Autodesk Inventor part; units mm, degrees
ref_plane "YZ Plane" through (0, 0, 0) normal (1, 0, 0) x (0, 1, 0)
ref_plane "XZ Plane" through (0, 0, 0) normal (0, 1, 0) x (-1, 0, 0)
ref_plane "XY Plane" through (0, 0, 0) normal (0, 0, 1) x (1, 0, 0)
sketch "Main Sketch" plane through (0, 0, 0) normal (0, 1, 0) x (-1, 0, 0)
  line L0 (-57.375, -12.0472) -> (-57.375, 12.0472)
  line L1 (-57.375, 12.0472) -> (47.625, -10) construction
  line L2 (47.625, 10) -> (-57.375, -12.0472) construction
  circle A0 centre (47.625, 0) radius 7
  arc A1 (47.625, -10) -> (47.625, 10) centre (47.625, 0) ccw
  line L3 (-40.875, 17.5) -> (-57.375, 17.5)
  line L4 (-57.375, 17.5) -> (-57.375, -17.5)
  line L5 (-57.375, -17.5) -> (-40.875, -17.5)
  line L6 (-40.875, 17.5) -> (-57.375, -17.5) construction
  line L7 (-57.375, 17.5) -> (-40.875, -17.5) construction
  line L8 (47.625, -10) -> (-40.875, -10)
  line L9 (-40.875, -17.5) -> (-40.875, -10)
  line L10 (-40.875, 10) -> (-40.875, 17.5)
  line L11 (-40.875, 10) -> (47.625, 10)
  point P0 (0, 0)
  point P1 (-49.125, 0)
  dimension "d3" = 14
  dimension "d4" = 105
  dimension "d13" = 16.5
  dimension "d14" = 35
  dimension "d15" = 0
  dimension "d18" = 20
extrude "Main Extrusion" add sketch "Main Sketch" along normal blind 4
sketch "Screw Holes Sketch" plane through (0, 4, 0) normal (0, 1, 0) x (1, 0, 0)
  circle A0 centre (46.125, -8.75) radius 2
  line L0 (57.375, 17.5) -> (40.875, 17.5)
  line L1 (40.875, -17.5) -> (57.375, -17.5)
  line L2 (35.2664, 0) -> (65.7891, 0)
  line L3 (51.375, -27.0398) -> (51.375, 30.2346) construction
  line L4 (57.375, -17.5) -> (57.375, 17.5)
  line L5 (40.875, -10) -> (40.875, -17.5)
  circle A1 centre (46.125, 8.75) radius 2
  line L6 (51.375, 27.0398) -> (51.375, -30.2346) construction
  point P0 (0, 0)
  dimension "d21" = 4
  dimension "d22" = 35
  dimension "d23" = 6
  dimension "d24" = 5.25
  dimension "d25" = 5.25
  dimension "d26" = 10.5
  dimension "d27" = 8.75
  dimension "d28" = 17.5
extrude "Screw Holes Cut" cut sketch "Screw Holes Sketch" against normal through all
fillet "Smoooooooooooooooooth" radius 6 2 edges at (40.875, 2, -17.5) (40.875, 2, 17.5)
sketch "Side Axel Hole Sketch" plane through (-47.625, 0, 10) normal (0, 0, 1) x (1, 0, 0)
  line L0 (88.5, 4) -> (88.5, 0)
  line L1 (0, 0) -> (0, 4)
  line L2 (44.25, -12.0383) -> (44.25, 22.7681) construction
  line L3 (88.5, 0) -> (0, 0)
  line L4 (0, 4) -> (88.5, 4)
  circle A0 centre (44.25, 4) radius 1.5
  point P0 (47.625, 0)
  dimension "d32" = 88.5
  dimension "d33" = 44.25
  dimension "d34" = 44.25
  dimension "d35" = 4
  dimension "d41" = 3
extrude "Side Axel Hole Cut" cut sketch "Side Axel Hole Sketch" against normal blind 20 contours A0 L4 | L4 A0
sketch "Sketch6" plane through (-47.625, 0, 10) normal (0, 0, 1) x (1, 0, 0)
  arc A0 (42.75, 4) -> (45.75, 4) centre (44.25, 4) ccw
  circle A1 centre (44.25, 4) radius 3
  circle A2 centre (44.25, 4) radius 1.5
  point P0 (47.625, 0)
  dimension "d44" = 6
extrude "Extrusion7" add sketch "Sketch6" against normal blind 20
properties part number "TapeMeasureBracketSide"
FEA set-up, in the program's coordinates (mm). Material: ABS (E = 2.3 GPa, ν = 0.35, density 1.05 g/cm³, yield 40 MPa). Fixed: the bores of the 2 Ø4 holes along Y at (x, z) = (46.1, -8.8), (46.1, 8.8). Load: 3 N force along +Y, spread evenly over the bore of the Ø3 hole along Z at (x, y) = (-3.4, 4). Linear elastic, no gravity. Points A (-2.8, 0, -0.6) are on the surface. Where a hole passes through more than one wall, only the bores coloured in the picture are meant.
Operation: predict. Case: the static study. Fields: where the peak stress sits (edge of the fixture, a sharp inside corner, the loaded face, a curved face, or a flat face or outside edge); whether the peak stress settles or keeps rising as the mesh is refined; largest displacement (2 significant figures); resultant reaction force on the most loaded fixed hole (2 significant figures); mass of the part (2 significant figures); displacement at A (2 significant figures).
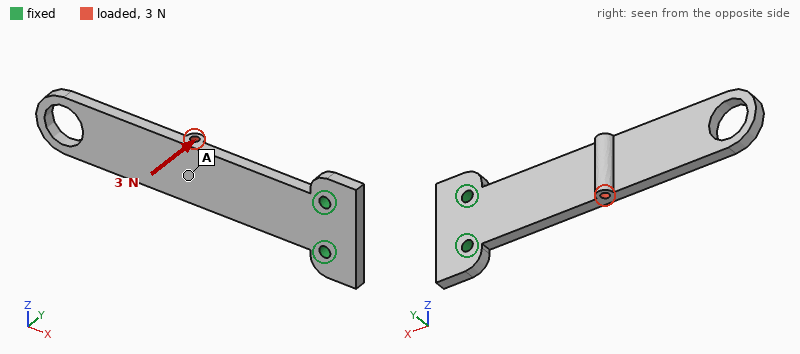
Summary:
edge of the fixture
keeps rising
1.2 mm
1.5 N
9.9 g
0.46 mm
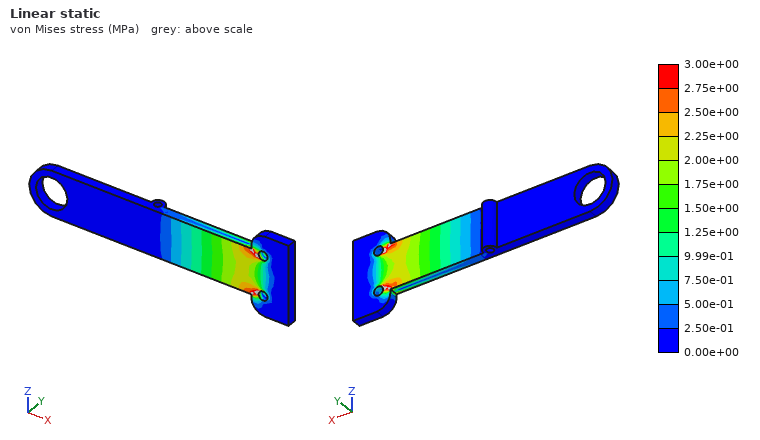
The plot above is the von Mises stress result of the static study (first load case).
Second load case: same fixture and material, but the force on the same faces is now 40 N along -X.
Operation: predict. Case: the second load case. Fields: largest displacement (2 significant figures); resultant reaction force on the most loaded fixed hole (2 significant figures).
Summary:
1.2 mm
21 N
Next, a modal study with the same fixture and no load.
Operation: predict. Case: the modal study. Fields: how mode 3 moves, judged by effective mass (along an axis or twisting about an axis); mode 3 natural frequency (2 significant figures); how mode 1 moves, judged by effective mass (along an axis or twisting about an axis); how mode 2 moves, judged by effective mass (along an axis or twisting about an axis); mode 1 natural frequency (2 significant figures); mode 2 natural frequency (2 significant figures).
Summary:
along Y
630 Hz
along Y
along Z
110 Hz
530 Hz
